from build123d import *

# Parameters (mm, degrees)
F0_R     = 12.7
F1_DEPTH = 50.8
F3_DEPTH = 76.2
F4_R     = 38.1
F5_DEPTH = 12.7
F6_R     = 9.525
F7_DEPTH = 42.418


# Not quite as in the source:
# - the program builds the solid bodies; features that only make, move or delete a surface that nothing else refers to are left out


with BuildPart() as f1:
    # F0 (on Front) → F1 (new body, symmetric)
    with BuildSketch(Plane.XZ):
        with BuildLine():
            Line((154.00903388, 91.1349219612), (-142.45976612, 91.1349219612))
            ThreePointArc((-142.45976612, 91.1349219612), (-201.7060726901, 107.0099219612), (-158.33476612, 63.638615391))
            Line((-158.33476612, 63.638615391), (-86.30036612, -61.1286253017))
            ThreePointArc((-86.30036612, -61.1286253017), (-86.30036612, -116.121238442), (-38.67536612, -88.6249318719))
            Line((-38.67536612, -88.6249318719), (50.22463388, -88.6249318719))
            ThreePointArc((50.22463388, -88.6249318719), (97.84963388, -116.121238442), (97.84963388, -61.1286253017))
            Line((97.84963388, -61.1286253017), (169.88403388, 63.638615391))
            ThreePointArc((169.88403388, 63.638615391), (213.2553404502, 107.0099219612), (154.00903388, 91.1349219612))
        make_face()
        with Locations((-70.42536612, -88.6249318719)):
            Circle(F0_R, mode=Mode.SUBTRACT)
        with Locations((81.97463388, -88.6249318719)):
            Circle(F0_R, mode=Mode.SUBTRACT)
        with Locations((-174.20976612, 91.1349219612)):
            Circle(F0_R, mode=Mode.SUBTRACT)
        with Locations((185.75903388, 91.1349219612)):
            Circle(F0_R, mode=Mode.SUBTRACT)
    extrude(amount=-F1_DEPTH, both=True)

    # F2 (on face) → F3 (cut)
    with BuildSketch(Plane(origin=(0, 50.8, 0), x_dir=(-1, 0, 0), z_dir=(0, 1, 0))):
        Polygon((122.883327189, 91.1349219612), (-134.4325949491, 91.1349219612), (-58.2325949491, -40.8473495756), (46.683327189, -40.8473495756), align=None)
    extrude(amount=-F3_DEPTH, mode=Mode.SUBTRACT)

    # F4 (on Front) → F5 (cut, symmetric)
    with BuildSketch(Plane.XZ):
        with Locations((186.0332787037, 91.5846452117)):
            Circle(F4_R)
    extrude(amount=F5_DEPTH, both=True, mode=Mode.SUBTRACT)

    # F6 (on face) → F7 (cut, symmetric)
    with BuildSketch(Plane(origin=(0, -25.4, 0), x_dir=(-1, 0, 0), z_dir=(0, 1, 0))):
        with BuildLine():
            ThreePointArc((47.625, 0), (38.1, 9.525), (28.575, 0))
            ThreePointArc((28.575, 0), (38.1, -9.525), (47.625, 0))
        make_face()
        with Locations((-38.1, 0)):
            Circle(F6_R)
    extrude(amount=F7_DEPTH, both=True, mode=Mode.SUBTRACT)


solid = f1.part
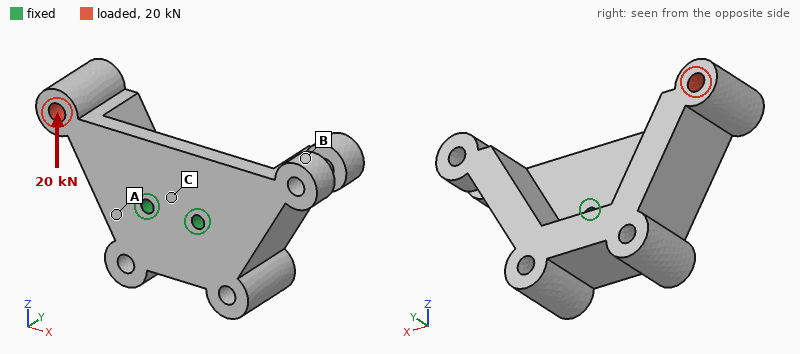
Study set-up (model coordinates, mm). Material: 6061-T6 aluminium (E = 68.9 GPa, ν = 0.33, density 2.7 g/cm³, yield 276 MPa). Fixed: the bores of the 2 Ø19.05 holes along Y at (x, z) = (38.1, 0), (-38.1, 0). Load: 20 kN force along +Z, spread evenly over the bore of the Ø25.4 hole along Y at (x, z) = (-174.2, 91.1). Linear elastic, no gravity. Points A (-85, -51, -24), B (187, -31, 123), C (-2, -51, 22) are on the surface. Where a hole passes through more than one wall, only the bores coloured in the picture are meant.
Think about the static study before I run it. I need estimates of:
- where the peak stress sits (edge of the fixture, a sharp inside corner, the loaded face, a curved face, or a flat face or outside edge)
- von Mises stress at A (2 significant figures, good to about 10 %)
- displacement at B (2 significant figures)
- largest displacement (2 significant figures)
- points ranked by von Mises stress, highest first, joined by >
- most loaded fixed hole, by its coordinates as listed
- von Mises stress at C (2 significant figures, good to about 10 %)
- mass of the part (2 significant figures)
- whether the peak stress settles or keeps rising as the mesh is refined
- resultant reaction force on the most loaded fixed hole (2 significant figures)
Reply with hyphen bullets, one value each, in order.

- edge of the fixture
- 12 MPa
- 0.11 mm
- 0.39 mm
- C > A > B
- (-38.1, 0)
- 20 MPa
- 9.5 kg
- keeps rising
- 48 kN
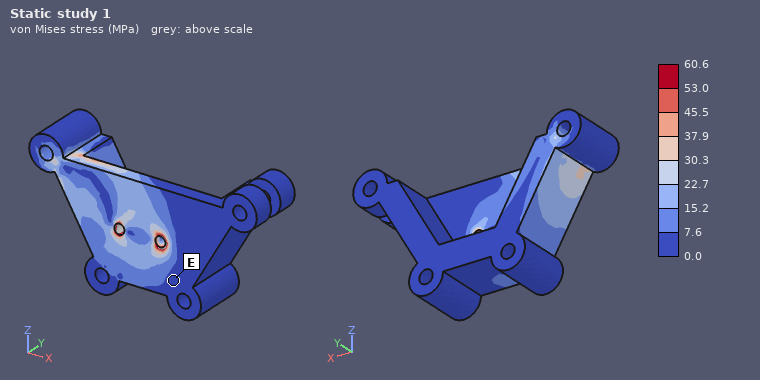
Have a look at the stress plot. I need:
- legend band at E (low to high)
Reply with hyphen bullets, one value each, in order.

- 0.0 to 7.6 MPa
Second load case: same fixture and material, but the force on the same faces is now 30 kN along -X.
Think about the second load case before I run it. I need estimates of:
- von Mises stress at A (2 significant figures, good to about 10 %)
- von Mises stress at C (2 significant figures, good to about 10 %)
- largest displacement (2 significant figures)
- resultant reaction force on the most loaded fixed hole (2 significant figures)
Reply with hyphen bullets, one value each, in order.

- 27 MPa
- 22 MPa
- 0.56 mm
- 35 kN
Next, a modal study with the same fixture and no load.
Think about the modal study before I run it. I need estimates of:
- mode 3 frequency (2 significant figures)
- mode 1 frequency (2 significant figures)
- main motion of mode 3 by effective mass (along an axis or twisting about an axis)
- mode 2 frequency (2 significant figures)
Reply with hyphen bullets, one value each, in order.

- 1100 Hz
- 610 Hz
- twisting about Y
- 760 Hz
